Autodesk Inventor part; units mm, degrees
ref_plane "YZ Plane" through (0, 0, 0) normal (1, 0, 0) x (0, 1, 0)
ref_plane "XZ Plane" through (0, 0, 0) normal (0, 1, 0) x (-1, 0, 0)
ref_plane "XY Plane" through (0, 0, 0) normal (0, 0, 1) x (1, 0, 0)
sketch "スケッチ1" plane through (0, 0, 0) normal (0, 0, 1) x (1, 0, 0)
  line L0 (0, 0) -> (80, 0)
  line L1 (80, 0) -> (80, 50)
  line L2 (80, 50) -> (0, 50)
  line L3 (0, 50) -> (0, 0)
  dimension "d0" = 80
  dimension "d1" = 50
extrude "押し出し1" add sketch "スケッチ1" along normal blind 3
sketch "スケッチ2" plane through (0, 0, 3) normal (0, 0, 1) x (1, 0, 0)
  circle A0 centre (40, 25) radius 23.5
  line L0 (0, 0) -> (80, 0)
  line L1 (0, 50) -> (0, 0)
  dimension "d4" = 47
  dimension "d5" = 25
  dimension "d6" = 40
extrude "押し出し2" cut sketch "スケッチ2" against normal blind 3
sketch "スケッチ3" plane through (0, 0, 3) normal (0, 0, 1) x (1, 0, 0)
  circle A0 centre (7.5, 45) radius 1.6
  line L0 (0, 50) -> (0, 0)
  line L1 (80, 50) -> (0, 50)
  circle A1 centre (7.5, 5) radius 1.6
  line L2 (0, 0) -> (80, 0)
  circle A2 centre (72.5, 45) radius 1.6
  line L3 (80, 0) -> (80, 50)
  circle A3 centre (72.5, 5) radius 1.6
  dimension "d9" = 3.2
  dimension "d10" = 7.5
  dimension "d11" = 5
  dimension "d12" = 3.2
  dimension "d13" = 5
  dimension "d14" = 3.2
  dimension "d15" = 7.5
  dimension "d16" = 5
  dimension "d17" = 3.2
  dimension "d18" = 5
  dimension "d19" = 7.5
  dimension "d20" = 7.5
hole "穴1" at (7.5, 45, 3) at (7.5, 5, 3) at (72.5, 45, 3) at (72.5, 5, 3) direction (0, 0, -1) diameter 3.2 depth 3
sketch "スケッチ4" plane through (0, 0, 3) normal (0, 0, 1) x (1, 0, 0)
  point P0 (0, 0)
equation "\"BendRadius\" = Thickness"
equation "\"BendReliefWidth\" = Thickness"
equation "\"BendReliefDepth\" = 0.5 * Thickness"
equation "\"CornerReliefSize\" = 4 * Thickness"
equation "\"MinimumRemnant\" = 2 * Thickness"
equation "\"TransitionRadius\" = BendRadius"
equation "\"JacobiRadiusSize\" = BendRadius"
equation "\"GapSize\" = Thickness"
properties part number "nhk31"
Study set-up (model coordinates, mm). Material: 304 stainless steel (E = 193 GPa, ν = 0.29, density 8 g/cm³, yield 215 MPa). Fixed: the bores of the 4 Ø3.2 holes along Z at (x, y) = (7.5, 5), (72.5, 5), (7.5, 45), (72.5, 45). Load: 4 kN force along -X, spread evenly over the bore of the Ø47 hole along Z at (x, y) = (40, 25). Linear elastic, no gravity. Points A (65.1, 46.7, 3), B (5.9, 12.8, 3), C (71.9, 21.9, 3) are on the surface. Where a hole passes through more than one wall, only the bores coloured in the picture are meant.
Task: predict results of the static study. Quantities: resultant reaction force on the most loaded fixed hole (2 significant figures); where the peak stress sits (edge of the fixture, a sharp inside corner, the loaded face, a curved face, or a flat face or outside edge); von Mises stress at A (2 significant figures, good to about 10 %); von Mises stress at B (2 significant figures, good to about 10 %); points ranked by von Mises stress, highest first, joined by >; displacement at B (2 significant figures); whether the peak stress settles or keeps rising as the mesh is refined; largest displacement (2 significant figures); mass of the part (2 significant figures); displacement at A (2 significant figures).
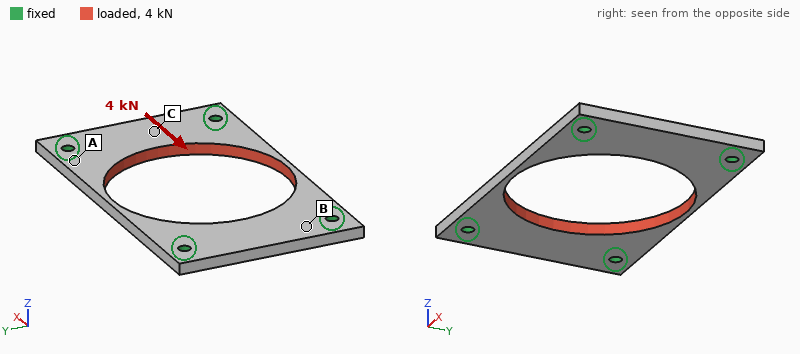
1.0 kN
edge of the fixture
25 MPa
14 MPa
A > B > C
2.1 µm
keeps rising
3.9 µm
54 g
1.1 µm
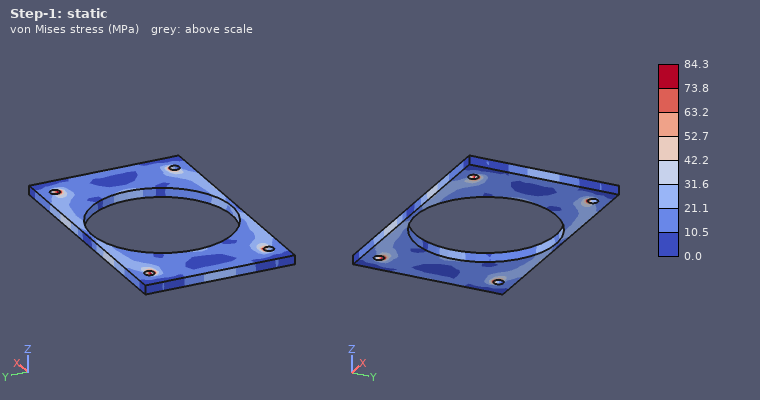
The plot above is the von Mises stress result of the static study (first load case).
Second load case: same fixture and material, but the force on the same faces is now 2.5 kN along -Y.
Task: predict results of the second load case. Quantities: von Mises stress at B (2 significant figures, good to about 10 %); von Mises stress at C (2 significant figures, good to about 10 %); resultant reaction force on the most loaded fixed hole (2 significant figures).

17 MPa
19 MPa
630 N
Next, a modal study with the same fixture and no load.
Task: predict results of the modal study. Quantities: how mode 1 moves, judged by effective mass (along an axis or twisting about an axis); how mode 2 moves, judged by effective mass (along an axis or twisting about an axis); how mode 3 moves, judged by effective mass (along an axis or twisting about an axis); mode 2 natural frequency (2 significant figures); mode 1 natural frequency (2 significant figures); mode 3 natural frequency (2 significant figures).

along Z
twisting about X
twisting about Y
5600 Hz
5400 Hz
8500 Hz
